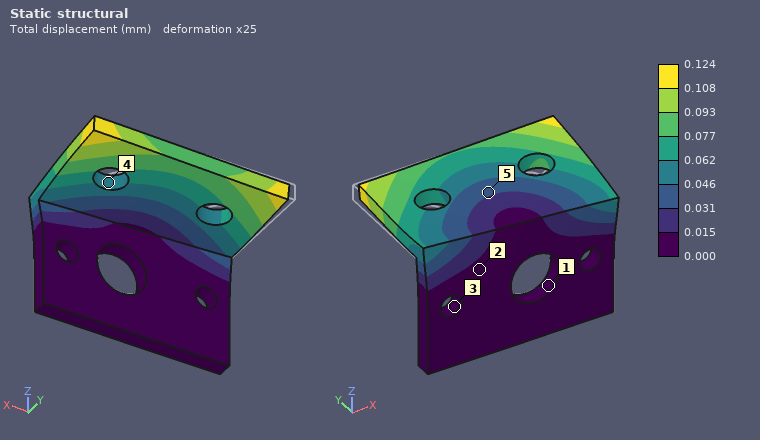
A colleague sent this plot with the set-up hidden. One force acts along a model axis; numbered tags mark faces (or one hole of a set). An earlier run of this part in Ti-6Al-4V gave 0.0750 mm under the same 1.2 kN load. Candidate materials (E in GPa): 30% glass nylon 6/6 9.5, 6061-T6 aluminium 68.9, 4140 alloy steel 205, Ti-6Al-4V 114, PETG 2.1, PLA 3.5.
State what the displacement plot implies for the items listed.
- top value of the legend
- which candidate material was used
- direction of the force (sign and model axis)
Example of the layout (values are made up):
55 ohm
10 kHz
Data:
0.124 mm
6061-T6 aluminium
+X
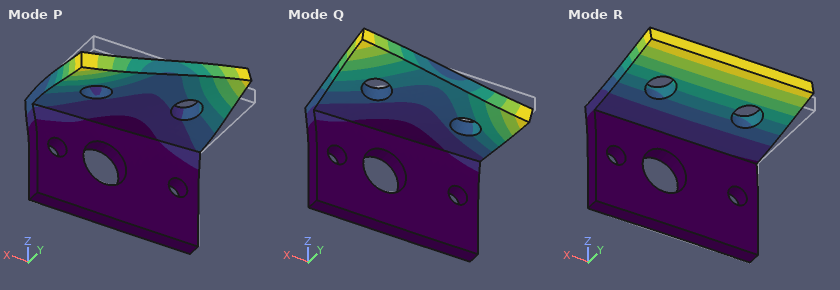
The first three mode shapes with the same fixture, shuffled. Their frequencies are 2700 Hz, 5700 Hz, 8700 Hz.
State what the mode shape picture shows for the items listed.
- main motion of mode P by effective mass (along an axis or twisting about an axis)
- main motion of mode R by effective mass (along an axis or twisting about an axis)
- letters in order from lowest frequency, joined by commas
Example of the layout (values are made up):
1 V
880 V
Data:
along X
along Z
R, Q, P
